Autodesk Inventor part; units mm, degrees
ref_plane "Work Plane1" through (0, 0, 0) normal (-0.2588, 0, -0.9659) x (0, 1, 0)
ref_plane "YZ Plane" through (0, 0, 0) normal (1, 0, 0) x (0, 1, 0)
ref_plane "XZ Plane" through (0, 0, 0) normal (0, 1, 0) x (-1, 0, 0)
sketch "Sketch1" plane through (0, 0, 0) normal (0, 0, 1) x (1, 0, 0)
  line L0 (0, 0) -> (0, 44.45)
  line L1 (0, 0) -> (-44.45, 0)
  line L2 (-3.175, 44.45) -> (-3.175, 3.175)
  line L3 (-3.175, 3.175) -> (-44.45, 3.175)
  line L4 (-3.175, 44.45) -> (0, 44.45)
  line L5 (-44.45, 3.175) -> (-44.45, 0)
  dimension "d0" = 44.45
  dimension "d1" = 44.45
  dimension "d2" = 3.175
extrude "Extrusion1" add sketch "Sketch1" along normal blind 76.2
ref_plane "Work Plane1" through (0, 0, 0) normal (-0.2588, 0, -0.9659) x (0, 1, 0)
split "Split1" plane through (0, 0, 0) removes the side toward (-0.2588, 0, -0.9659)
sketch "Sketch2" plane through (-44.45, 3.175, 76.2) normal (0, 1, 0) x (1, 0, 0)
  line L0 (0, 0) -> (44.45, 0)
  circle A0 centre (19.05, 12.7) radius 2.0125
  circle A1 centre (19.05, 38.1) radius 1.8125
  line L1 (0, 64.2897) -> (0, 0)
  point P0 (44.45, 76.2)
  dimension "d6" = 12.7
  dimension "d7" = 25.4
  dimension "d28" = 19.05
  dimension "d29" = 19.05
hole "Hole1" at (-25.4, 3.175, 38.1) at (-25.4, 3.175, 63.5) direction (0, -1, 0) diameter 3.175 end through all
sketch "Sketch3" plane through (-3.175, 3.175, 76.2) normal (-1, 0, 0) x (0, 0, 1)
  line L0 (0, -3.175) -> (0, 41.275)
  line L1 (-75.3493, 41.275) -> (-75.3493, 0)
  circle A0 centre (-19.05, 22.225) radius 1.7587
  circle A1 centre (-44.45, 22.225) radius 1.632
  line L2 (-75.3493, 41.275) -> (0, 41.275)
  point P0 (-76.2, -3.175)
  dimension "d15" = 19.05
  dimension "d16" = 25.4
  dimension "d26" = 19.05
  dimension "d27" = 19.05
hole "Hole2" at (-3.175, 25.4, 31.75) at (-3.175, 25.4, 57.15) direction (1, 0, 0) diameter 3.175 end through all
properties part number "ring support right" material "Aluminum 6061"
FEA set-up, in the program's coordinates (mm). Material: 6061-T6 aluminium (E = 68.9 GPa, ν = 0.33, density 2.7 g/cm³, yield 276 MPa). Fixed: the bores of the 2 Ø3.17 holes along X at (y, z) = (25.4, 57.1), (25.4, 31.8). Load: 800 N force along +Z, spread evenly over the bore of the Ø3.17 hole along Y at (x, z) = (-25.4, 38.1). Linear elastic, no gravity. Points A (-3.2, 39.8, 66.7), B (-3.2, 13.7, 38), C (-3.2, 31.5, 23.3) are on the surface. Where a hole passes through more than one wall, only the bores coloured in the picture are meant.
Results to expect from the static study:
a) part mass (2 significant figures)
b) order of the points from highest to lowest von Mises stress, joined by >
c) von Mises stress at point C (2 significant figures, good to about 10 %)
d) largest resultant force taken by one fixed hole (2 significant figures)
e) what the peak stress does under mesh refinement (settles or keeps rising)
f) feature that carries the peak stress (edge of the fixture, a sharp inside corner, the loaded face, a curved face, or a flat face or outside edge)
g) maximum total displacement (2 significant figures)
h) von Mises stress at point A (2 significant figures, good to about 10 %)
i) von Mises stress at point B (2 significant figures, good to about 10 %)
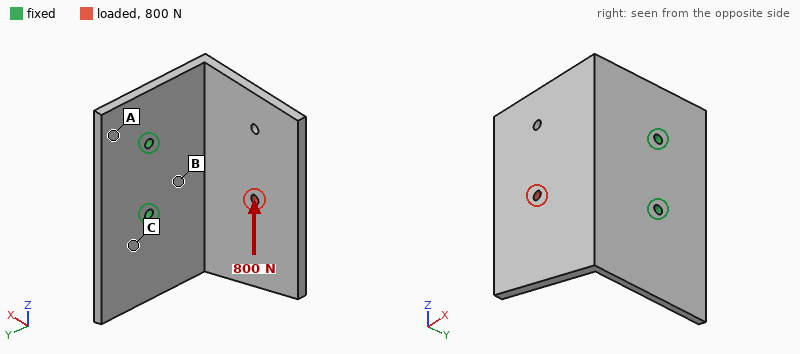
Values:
53 g
B > C > A
61 MPa
990 N
keeps rising
edge of the fixture
0.62 mm
24 MPa
92 MPa
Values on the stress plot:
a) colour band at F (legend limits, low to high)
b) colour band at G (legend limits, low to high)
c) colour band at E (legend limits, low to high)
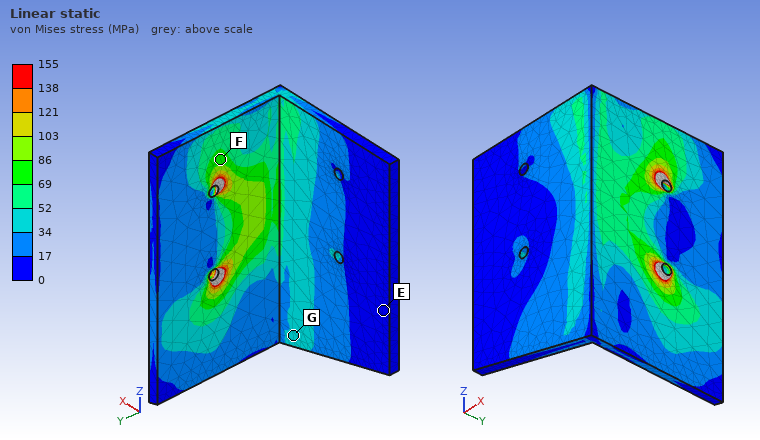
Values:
69 to 86 MPa
34 to 52 MPa
0 to 17 MPa
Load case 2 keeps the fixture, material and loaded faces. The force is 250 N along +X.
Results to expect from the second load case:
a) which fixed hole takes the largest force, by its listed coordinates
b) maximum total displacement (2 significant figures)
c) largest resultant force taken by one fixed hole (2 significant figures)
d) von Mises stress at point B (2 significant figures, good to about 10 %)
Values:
(25.4, 31.8)
0.33 mm
170 N
29 MPa
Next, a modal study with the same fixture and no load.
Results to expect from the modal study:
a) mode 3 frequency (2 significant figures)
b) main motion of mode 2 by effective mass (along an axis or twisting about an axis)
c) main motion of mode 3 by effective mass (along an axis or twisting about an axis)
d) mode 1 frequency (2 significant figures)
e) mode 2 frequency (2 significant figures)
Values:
2200 Hz
along Z
along X
730 Hz
1200 Hz
